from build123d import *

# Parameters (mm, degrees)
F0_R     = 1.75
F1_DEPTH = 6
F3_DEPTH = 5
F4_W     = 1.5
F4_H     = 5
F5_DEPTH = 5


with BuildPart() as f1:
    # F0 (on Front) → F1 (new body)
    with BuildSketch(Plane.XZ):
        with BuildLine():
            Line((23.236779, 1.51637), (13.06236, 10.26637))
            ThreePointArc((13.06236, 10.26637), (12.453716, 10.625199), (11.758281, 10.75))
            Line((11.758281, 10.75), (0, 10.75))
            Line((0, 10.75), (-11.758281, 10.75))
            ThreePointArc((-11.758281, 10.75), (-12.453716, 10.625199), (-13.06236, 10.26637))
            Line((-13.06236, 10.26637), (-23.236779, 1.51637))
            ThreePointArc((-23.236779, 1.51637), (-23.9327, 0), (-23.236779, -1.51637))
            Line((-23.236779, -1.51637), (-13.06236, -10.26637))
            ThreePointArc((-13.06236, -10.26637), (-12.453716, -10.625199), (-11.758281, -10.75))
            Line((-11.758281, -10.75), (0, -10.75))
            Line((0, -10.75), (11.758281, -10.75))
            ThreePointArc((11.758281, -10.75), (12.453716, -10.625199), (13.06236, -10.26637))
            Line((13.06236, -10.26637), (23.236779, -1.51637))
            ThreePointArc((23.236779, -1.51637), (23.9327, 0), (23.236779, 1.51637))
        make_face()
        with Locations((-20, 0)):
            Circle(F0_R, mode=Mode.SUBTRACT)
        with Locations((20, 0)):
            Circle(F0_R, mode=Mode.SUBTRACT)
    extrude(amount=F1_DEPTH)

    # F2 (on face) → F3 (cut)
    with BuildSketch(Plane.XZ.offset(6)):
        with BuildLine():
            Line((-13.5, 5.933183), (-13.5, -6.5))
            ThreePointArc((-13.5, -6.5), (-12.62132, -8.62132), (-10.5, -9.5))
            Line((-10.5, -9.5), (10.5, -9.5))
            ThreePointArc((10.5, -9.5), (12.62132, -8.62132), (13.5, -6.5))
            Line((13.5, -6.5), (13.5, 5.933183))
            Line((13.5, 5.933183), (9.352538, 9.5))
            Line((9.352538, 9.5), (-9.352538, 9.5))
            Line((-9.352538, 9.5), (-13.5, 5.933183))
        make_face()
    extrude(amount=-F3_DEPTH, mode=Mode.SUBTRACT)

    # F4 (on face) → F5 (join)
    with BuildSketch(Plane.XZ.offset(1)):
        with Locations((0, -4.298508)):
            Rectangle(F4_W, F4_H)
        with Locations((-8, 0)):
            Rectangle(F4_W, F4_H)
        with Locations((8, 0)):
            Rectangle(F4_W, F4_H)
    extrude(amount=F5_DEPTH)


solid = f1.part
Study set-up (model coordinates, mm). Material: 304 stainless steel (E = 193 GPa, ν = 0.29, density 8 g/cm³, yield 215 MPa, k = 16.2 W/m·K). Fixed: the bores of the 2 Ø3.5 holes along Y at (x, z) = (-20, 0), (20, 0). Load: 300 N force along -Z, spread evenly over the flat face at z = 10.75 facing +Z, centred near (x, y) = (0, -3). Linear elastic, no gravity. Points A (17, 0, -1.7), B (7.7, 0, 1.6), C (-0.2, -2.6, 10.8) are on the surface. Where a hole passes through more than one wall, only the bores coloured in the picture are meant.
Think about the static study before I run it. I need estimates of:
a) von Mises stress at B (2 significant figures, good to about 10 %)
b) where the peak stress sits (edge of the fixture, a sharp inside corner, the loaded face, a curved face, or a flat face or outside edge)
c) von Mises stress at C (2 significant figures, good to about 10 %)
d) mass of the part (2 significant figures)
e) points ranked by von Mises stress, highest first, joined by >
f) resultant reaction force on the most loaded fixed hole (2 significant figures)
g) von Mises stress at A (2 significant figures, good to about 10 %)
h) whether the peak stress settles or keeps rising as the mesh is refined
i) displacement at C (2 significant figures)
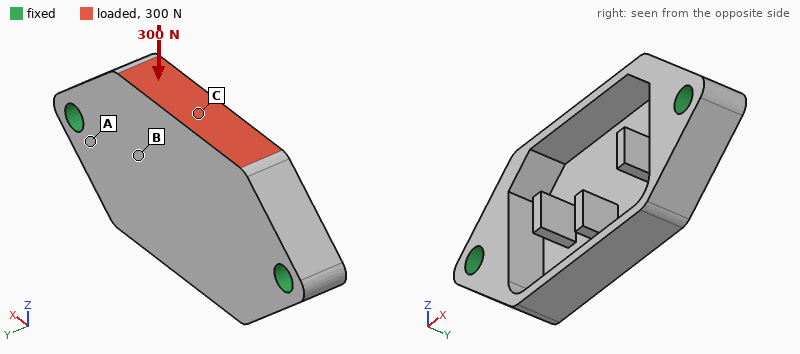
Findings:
12 MPa
a sharp inside corner
32 MPa
19 g
C > B > A
170 N
5.0 MPa
keeps rising
7.2 µm
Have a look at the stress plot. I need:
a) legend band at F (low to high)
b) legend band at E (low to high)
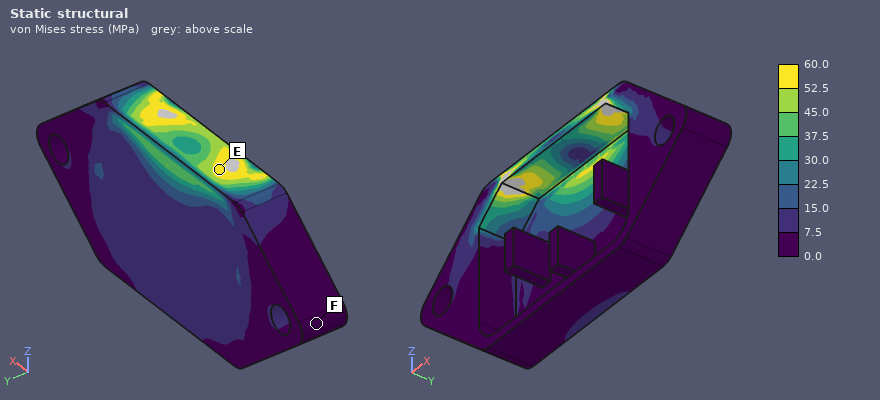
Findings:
0.0 to 7.5 MPa
52.5 to 60.0 MPa
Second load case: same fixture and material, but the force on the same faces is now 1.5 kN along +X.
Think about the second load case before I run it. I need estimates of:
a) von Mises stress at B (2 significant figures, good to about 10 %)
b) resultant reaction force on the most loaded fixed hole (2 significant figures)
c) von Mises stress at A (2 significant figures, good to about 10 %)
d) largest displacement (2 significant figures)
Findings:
32 MPa
830 N
15 MPa
11 µm
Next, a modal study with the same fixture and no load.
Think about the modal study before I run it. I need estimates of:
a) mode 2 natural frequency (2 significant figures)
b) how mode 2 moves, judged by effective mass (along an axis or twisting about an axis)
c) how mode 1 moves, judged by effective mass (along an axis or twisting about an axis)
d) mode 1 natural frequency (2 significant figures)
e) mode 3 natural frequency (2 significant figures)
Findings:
16 kHz
twisting about X
along Y
10000 Hz
19 kHz
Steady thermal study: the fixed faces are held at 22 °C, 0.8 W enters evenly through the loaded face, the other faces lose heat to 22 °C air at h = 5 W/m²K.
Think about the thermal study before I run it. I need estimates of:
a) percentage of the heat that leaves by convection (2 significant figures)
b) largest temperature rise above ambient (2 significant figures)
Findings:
6.7 %
16 K
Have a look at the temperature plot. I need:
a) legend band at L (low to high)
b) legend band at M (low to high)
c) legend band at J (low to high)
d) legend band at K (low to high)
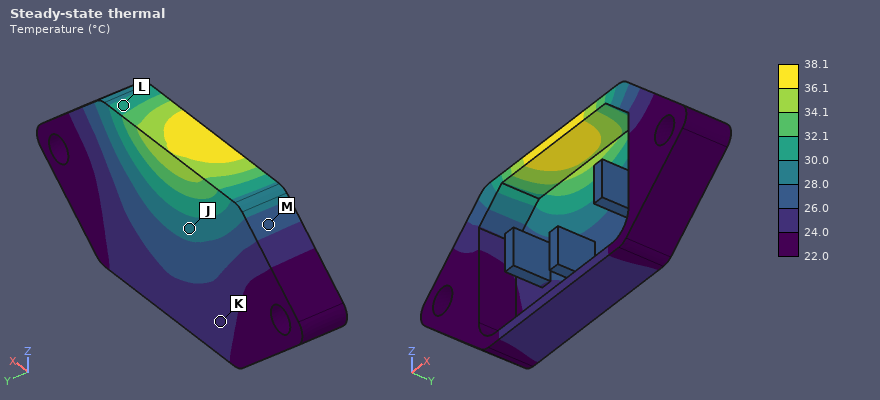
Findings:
30.0 to 32.1 °C
26.0 to 28.0 °C
28.0 to 30.0 °C
24.0 to 26.0 °C
